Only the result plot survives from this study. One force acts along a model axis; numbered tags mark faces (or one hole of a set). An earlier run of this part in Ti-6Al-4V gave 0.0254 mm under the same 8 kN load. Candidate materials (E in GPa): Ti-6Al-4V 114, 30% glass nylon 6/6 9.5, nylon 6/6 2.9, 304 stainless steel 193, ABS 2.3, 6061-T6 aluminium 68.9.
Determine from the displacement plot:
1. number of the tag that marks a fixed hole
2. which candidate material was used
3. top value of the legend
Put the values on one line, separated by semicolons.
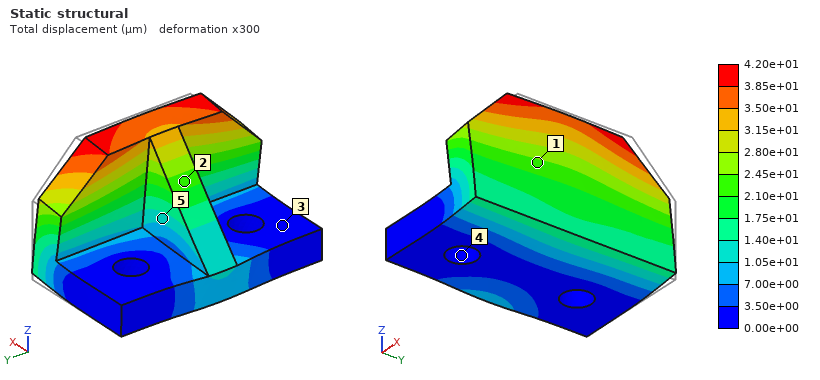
4; 6061-T6 aluminium; 4.20e+01 µm
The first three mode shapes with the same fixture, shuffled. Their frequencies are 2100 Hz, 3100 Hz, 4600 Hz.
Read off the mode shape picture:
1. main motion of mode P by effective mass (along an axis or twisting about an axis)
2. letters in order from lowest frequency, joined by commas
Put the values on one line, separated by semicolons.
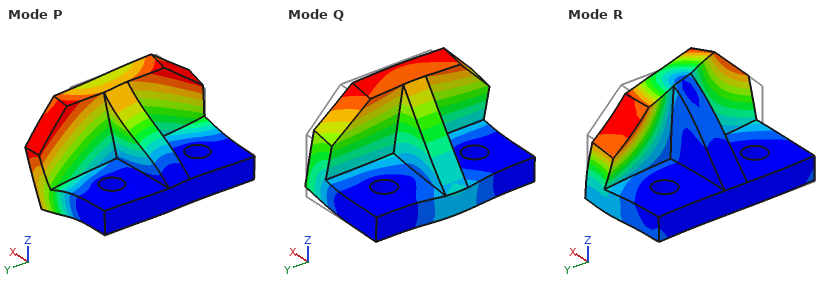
along Y; Q, P, R
